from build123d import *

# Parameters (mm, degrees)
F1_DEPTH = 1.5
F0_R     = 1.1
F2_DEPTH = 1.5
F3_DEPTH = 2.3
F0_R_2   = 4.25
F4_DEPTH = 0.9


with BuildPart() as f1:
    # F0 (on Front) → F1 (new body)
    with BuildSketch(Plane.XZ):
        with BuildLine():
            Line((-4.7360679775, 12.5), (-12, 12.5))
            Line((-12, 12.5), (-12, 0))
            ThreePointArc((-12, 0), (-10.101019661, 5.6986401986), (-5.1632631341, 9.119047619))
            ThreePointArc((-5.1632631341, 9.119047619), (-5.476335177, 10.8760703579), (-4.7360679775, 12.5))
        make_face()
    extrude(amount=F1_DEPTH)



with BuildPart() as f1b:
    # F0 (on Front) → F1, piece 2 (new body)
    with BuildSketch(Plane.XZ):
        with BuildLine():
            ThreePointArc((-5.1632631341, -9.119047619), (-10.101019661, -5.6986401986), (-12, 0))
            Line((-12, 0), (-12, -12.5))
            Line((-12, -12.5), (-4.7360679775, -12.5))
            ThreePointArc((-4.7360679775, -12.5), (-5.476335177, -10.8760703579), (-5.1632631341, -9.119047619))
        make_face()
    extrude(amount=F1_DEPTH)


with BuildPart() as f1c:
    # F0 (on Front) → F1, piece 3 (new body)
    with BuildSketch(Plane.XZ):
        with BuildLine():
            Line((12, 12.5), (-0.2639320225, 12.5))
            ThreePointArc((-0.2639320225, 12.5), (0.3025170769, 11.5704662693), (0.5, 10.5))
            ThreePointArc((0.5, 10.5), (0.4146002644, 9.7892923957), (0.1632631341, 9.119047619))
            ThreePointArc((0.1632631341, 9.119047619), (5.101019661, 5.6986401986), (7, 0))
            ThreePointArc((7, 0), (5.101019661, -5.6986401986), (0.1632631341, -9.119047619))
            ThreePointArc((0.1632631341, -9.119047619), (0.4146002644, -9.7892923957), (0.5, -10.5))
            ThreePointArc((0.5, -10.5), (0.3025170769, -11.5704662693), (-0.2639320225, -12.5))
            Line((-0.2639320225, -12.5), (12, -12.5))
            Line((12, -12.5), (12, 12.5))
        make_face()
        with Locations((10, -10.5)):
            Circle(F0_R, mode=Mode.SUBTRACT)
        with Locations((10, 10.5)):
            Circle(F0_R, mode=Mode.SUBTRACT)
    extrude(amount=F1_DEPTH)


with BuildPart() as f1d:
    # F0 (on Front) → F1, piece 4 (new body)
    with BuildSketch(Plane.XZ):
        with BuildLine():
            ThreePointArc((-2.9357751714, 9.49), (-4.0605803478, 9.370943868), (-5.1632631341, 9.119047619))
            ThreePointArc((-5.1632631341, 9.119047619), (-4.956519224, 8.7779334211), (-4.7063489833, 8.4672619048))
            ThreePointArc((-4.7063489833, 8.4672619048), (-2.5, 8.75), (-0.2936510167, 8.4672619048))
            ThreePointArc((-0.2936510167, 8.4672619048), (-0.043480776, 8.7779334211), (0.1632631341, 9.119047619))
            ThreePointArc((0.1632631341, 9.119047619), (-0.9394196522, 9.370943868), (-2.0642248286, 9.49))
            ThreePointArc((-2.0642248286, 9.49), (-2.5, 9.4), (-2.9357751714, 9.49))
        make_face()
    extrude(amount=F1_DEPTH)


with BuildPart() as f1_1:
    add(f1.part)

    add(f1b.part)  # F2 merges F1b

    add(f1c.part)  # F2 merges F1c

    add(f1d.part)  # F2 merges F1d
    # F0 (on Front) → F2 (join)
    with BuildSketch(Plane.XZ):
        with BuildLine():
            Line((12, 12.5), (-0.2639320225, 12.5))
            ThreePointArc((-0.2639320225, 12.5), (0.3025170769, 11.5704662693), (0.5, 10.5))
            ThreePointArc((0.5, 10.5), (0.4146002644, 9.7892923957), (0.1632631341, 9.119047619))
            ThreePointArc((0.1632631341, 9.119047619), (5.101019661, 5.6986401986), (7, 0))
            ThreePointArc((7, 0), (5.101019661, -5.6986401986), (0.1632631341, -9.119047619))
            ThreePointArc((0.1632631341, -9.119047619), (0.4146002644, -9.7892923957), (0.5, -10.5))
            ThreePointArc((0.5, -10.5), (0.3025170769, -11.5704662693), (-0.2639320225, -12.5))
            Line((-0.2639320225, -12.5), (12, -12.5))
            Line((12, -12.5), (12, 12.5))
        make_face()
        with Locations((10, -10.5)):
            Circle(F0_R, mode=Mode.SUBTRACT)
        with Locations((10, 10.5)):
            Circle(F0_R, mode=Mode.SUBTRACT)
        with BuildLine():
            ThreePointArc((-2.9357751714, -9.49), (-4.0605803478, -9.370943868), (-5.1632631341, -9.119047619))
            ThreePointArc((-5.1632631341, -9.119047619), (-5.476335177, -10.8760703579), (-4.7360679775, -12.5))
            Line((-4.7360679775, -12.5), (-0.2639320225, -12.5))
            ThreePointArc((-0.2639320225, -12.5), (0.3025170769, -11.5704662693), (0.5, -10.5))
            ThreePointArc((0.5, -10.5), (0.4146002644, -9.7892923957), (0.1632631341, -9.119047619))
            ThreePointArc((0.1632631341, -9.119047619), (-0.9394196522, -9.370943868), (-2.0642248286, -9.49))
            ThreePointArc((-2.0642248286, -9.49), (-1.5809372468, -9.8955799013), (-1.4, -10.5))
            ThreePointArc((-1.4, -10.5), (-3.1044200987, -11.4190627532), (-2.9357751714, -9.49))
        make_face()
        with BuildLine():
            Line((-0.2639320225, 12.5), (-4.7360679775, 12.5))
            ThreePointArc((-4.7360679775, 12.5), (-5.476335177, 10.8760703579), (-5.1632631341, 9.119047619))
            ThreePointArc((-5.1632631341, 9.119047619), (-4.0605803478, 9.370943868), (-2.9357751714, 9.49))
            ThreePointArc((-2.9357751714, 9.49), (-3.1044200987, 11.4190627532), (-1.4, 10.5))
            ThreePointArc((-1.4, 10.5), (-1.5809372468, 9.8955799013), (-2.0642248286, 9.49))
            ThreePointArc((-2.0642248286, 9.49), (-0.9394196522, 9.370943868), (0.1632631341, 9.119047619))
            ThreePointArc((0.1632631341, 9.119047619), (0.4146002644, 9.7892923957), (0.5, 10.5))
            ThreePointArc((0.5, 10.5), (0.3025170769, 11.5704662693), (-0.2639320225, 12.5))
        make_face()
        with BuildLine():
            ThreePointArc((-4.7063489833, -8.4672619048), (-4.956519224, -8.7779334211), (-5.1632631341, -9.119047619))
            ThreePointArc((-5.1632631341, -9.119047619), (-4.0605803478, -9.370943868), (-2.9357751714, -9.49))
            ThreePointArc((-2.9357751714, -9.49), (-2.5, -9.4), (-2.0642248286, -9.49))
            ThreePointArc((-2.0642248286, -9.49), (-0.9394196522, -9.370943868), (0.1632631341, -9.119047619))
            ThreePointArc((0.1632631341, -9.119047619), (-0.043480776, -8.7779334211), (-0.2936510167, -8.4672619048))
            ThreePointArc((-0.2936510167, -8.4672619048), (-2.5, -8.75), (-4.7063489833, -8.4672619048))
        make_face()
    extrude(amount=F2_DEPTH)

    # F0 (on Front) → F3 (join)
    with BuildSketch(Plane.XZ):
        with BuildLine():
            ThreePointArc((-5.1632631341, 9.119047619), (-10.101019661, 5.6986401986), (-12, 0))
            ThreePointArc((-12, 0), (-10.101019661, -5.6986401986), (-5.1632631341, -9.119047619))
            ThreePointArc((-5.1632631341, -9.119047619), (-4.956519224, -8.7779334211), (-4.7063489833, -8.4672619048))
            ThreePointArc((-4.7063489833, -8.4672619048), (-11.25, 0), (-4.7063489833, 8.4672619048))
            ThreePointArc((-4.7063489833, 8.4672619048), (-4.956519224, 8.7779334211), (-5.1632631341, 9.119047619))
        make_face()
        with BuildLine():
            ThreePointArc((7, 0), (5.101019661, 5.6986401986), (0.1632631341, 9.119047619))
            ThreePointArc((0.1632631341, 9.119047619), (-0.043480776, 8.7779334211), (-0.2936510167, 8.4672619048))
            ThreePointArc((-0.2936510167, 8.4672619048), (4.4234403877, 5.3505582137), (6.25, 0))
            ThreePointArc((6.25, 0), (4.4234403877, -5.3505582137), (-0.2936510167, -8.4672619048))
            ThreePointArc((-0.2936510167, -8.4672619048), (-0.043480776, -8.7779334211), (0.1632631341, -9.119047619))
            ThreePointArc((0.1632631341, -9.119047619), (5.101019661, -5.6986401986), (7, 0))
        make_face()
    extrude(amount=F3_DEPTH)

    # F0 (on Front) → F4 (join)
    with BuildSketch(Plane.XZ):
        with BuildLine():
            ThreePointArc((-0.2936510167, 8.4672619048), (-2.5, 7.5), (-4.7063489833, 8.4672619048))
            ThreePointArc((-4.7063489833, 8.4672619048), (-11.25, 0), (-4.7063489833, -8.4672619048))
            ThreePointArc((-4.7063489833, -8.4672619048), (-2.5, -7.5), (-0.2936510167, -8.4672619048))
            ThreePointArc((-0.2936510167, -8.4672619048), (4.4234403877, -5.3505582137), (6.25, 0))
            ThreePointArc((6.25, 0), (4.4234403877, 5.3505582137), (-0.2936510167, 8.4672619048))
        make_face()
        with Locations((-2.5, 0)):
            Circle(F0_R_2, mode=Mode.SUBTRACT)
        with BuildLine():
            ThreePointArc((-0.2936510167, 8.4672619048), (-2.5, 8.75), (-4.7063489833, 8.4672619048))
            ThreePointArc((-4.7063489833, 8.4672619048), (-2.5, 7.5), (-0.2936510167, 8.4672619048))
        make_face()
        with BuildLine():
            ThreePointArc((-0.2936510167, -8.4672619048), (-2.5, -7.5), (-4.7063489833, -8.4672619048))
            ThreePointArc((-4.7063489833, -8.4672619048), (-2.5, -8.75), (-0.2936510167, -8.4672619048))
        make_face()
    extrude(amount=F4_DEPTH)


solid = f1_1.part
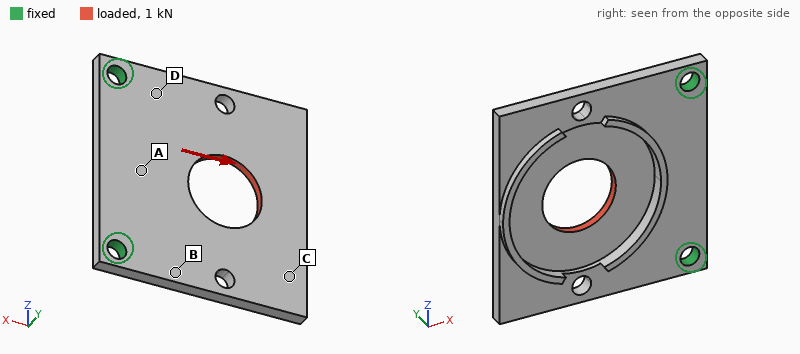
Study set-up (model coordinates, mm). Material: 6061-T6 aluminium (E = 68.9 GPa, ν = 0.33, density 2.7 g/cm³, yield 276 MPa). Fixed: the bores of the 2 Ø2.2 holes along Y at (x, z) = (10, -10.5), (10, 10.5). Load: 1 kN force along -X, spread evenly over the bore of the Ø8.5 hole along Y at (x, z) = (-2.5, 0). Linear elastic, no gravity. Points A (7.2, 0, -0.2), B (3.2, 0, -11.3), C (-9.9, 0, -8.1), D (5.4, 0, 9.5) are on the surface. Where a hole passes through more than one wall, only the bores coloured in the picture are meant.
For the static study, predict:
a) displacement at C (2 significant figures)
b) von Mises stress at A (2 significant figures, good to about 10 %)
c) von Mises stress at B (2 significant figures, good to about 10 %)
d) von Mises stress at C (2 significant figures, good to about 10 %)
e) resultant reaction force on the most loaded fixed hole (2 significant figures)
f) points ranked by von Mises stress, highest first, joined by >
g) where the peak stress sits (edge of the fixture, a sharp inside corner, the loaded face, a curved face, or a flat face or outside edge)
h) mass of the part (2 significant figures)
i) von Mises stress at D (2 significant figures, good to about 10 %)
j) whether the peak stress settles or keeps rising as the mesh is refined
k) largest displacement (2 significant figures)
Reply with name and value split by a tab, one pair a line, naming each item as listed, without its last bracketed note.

displacement at C	0.12 mm
von Mises stress at A	26 MPa
von Mises stress at B	67 MPa
von Mises stress at C	12 MPa
resultant reaction force on the most loaded fixed hole	530 N
points ranked by von Mises stress, highest first, joined by >	D > B > A > C
where the peak stress sits	edge of the fixture
mass of the part	1.9 g
von Mises stress at D	83 MPa
whether the peak stress settles or keeps rising as the mesh is refined	keeps rising
largest displacement	0.13 mm
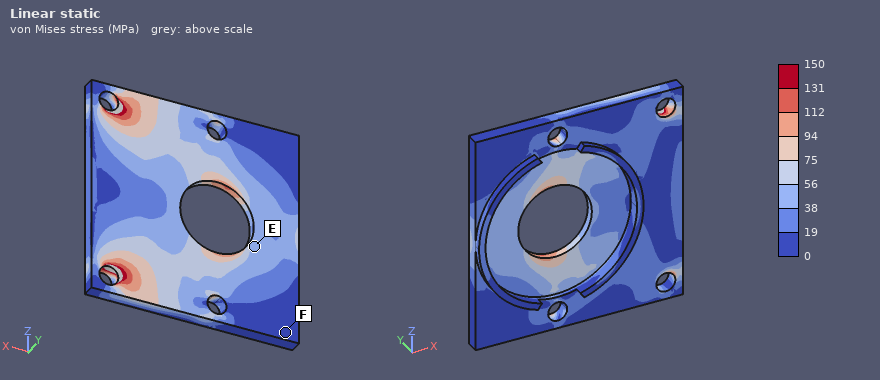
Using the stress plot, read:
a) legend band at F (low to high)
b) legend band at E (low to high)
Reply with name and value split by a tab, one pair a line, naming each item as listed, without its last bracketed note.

legend band at F	0 to 19 MPa
legend band at E	38 to 56 MPa
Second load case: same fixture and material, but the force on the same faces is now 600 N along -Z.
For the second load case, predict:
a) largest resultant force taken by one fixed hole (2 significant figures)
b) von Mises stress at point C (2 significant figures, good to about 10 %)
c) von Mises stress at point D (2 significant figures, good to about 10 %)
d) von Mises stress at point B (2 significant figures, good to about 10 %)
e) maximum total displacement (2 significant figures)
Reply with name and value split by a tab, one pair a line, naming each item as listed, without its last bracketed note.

largest resultant force taken by one fixed hole	450 N
von Mises stress at point C	15 MPa
von Mises stress at point D	44 MPa
von Mises stress at point B	42 MPa
maximum total displacement	33 µm
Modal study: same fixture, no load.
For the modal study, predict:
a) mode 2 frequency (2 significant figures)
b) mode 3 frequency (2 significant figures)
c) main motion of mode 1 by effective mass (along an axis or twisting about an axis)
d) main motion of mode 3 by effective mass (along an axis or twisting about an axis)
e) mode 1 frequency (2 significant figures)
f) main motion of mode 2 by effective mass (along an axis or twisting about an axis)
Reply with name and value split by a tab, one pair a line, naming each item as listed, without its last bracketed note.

mode 2 frequency	4900 Hz
mode 3 frequency	12 kHz
main motion of mode 1 by effective mass	along Y
main motion of mode 3 by effective mass	along Y
mode 1 frequency	2200 Hz
main motion of mode 2 by effective mass	twisting about X
